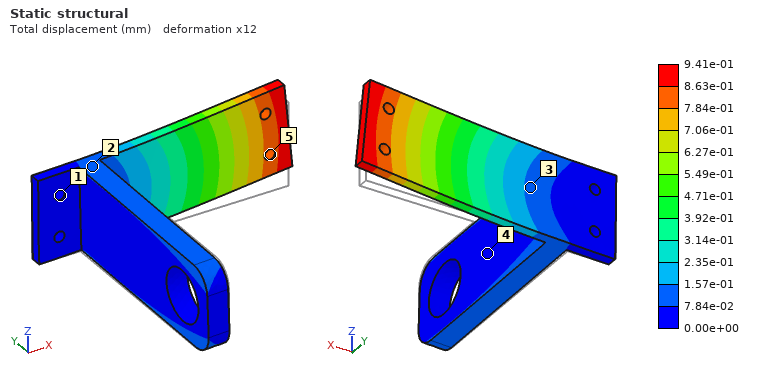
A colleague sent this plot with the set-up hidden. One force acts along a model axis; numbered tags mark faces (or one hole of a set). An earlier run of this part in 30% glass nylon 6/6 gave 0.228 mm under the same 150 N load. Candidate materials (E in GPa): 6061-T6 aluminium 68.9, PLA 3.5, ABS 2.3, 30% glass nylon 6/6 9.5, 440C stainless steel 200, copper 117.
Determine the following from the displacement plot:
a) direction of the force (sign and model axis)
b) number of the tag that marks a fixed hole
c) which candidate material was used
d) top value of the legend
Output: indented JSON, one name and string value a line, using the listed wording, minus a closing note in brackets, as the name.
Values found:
{
  "direction of the force": "+Z",
  "number of the tag that marks a fixed hole": "1",
  "which candidate material was used": "ABS",
  "top value of the legend": "9.41e-01 mm"
}
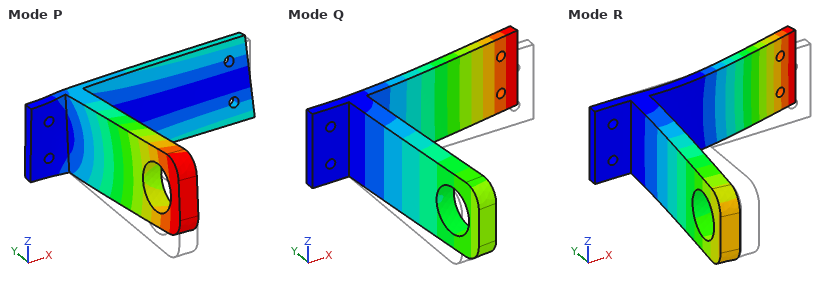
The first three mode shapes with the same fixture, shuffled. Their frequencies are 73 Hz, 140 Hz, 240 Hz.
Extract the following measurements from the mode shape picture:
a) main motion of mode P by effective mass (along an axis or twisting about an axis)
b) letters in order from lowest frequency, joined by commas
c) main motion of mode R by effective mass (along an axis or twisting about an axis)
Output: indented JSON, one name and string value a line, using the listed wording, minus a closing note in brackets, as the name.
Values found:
{
  "main motion of mode P by effective mass": "along Z",
  "letters in order from lowest frequency, joined by commas": "Q, R, P",
  "main motion of mode R by effective mass": "along X"
}
